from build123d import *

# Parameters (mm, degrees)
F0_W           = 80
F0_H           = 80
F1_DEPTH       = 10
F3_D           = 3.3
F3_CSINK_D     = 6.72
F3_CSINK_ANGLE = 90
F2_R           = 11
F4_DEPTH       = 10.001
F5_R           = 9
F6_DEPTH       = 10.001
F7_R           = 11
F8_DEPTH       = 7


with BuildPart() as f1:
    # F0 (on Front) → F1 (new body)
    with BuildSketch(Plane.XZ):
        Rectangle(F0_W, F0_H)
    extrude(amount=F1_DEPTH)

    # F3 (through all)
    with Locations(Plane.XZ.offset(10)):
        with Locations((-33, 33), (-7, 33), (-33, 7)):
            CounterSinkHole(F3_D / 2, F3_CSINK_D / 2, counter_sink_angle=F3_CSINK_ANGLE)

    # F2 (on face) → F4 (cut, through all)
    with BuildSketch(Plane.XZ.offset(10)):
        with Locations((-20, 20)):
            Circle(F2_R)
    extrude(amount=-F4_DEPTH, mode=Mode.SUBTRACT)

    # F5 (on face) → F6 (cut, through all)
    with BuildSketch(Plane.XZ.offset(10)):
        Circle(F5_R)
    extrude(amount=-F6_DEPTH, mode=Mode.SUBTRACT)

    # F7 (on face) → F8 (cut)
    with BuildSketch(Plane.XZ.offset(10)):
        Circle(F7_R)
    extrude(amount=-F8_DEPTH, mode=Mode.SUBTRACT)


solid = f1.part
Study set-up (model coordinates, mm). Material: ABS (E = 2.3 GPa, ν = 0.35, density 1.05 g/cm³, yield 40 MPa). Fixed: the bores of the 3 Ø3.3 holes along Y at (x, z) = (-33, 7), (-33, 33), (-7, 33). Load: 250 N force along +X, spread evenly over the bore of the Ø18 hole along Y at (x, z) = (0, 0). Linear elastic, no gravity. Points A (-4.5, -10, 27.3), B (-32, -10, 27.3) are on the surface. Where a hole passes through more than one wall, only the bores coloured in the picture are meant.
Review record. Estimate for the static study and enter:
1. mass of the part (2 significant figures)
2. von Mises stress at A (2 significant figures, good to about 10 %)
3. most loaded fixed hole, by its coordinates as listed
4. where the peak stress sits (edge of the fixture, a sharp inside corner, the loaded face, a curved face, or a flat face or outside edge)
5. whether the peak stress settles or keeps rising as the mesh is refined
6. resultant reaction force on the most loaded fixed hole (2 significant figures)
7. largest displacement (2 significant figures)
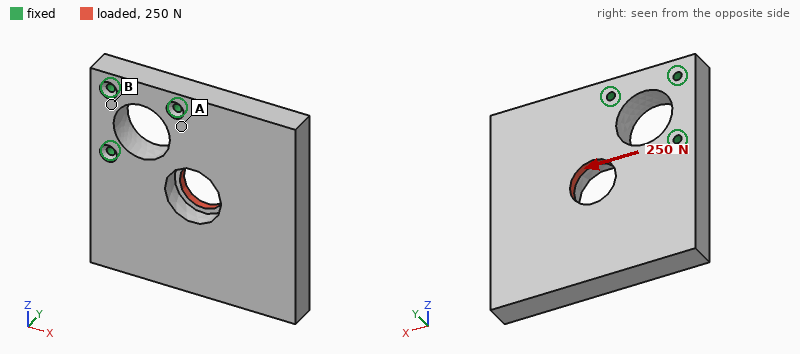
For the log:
59 g
1.1 MPa
(-33, 7)
edge of the fixture
keeps rising
230 N
0.17 mm
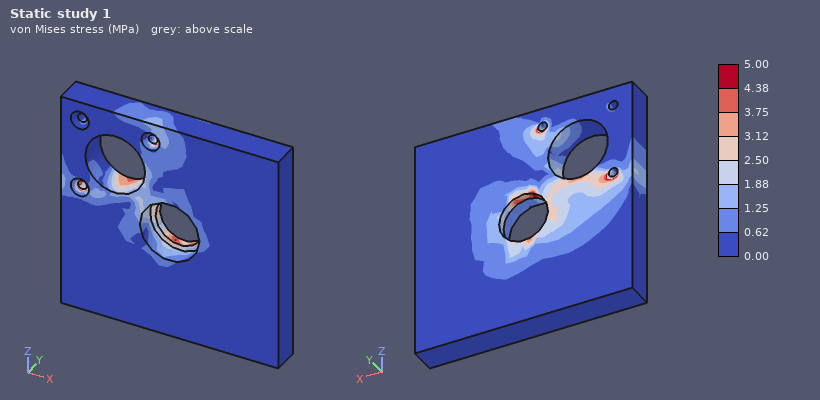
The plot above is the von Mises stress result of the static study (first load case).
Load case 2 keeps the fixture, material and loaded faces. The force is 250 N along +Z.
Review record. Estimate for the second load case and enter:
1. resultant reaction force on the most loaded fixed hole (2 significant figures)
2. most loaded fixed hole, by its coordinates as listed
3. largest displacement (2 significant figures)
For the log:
230 N
(-7, 33)
0.17 mm
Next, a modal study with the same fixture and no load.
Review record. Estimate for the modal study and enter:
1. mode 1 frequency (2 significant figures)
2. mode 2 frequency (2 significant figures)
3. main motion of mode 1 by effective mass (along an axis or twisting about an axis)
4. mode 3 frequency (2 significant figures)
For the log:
350 Hz
820 Hz
along Y
1100 Hz
